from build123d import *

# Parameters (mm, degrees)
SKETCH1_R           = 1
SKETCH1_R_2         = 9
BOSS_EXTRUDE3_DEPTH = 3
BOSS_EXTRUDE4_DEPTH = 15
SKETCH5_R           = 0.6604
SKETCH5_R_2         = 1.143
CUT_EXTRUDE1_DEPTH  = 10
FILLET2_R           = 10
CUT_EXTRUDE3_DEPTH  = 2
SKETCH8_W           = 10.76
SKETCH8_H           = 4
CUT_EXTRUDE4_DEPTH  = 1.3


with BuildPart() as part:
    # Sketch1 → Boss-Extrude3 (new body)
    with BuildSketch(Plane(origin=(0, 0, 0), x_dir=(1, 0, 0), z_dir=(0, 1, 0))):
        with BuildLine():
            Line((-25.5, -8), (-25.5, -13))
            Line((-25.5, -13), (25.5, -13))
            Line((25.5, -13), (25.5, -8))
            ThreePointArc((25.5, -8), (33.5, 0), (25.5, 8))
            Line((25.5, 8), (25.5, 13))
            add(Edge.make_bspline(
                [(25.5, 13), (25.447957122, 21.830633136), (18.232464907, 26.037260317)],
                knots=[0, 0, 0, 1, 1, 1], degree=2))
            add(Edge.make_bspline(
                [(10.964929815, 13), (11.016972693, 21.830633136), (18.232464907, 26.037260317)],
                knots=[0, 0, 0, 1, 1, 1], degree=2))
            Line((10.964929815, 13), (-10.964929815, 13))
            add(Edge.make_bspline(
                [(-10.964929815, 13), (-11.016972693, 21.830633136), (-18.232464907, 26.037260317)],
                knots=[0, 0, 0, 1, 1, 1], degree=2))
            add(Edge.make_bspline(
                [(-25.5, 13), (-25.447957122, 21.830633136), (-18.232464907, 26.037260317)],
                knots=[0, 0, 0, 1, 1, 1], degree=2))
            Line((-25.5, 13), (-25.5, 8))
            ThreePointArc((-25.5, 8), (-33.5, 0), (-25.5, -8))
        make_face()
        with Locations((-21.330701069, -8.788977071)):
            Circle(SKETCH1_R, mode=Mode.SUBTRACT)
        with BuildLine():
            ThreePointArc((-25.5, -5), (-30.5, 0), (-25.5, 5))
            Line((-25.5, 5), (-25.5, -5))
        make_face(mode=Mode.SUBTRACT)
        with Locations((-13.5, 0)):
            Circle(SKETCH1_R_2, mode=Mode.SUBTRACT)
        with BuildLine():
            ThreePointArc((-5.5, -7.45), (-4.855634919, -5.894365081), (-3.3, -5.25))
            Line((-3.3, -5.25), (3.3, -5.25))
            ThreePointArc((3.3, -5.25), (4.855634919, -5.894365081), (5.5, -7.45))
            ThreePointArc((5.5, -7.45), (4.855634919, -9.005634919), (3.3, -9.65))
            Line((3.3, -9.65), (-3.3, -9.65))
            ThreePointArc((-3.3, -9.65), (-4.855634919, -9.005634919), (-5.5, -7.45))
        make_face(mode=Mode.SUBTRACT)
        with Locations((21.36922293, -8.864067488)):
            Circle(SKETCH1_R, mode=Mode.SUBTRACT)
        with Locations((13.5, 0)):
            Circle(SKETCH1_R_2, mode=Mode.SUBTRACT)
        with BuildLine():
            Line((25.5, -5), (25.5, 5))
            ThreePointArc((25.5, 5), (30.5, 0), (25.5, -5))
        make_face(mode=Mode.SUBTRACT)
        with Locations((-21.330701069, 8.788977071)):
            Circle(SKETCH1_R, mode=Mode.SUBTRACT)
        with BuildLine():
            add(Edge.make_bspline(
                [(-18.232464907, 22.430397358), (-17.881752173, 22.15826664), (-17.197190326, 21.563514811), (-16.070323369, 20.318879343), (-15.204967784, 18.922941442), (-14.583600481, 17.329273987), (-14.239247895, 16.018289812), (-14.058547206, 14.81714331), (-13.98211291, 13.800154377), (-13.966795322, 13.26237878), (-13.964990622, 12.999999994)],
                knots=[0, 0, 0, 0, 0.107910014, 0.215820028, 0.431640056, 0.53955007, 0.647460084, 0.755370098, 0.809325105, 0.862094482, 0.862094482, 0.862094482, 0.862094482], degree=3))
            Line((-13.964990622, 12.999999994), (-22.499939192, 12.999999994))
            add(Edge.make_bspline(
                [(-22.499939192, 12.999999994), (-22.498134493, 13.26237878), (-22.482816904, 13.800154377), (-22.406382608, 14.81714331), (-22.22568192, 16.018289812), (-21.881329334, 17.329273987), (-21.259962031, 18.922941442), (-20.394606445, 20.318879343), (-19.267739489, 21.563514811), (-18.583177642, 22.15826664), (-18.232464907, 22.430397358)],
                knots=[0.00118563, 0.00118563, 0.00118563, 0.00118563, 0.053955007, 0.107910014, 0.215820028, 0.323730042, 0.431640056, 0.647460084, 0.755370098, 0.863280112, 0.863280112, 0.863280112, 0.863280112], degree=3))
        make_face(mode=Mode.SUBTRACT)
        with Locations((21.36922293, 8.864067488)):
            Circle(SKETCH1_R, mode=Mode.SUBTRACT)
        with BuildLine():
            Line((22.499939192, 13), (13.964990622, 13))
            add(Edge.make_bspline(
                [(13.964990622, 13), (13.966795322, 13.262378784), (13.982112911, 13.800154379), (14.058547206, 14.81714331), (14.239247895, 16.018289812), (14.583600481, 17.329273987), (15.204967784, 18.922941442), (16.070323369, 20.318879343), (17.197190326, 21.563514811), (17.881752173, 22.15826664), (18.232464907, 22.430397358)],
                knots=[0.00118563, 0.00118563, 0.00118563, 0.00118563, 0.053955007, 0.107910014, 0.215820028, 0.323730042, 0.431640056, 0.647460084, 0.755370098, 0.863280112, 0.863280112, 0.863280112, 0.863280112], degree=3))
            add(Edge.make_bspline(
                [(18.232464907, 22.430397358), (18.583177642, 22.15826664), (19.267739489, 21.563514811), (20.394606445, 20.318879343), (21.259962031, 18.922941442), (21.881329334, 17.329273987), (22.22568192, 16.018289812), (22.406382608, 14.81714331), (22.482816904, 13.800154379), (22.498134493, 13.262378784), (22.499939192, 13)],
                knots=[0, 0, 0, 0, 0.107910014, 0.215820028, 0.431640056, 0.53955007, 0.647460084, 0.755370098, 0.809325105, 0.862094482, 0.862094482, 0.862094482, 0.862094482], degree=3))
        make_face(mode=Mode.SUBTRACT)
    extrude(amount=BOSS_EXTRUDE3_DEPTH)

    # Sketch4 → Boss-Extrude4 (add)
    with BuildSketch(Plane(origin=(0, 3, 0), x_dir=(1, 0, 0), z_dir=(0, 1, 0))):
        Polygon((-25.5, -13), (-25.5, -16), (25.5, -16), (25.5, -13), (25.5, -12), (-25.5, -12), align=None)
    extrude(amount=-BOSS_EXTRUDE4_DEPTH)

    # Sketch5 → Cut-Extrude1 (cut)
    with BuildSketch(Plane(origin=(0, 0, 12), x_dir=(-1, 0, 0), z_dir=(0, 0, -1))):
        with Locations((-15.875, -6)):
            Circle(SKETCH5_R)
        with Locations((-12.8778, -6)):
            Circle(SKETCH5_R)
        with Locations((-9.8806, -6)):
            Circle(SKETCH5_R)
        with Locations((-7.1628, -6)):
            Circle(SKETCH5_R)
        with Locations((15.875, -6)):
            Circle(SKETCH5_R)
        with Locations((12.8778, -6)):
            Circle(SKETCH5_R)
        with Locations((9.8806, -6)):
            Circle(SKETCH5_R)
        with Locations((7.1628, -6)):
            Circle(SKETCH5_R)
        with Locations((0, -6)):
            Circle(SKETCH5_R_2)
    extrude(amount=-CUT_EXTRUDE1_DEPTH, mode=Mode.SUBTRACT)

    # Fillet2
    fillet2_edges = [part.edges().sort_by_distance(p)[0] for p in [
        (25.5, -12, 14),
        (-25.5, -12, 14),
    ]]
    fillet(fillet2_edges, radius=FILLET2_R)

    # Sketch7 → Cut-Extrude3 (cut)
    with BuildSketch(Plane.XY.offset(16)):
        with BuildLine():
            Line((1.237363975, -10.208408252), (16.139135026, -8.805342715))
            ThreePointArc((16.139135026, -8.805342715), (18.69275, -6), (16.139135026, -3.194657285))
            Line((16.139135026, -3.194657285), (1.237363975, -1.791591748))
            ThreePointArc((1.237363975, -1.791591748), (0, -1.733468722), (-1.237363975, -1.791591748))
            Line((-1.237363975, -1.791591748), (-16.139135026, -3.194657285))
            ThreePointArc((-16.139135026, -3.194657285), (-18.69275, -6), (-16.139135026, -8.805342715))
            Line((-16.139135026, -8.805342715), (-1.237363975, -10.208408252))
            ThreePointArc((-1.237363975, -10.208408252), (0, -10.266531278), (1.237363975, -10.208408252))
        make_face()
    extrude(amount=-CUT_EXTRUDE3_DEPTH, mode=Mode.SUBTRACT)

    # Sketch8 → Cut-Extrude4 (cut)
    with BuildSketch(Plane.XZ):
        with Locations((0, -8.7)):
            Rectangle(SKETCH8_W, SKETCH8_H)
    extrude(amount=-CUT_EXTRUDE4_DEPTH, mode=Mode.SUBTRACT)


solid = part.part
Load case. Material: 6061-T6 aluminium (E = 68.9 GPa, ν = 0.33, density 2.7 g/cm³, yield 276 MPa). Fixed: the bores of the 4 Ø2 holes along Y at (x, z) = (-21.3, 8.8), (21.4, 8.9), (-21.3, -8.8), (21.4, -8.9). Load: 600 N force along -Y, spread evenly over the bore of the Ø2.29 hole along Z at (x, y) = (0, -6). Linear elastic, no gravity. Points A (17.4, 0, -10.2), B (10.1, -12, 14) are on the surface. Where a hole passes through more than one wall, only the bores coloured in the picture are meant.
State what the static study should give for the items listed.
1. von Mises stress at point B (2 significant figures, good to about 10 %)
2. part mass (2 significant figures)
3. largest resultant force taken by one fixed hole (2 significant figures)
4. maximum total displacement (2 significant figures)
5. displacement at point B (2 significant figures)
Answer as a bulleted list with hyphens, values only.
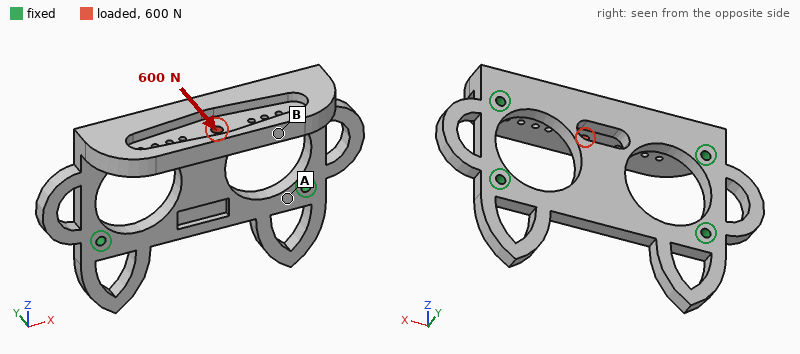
- 17 MPa
- 14 g
- 340 N
- 44 µm
- 35 µm
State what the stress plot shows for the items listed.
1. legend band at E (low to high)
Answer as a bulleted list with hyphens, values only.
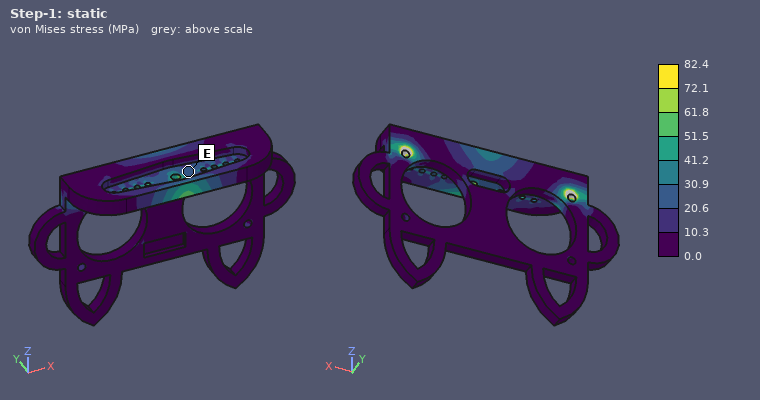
- 20.6 to 30.9 MPa
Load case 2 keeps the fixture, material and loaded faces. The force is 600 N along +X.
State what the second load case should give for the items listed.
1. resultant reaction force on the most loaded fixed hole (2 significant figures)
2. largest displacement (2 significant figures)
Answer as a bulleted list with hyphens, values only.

- 300 N
- 9.0 µm
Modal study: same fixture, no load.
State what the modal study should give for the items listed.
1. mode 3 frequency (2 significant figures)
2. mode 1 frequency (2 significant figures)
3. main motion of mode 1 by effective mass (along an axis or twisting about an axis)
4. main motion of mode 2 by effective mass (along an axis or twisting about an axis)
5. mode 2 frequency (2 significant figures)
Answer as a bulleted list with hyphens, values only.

- 8700 Hz
- 5900 Hz
- along Z
- along Y
- 7400 Hz
